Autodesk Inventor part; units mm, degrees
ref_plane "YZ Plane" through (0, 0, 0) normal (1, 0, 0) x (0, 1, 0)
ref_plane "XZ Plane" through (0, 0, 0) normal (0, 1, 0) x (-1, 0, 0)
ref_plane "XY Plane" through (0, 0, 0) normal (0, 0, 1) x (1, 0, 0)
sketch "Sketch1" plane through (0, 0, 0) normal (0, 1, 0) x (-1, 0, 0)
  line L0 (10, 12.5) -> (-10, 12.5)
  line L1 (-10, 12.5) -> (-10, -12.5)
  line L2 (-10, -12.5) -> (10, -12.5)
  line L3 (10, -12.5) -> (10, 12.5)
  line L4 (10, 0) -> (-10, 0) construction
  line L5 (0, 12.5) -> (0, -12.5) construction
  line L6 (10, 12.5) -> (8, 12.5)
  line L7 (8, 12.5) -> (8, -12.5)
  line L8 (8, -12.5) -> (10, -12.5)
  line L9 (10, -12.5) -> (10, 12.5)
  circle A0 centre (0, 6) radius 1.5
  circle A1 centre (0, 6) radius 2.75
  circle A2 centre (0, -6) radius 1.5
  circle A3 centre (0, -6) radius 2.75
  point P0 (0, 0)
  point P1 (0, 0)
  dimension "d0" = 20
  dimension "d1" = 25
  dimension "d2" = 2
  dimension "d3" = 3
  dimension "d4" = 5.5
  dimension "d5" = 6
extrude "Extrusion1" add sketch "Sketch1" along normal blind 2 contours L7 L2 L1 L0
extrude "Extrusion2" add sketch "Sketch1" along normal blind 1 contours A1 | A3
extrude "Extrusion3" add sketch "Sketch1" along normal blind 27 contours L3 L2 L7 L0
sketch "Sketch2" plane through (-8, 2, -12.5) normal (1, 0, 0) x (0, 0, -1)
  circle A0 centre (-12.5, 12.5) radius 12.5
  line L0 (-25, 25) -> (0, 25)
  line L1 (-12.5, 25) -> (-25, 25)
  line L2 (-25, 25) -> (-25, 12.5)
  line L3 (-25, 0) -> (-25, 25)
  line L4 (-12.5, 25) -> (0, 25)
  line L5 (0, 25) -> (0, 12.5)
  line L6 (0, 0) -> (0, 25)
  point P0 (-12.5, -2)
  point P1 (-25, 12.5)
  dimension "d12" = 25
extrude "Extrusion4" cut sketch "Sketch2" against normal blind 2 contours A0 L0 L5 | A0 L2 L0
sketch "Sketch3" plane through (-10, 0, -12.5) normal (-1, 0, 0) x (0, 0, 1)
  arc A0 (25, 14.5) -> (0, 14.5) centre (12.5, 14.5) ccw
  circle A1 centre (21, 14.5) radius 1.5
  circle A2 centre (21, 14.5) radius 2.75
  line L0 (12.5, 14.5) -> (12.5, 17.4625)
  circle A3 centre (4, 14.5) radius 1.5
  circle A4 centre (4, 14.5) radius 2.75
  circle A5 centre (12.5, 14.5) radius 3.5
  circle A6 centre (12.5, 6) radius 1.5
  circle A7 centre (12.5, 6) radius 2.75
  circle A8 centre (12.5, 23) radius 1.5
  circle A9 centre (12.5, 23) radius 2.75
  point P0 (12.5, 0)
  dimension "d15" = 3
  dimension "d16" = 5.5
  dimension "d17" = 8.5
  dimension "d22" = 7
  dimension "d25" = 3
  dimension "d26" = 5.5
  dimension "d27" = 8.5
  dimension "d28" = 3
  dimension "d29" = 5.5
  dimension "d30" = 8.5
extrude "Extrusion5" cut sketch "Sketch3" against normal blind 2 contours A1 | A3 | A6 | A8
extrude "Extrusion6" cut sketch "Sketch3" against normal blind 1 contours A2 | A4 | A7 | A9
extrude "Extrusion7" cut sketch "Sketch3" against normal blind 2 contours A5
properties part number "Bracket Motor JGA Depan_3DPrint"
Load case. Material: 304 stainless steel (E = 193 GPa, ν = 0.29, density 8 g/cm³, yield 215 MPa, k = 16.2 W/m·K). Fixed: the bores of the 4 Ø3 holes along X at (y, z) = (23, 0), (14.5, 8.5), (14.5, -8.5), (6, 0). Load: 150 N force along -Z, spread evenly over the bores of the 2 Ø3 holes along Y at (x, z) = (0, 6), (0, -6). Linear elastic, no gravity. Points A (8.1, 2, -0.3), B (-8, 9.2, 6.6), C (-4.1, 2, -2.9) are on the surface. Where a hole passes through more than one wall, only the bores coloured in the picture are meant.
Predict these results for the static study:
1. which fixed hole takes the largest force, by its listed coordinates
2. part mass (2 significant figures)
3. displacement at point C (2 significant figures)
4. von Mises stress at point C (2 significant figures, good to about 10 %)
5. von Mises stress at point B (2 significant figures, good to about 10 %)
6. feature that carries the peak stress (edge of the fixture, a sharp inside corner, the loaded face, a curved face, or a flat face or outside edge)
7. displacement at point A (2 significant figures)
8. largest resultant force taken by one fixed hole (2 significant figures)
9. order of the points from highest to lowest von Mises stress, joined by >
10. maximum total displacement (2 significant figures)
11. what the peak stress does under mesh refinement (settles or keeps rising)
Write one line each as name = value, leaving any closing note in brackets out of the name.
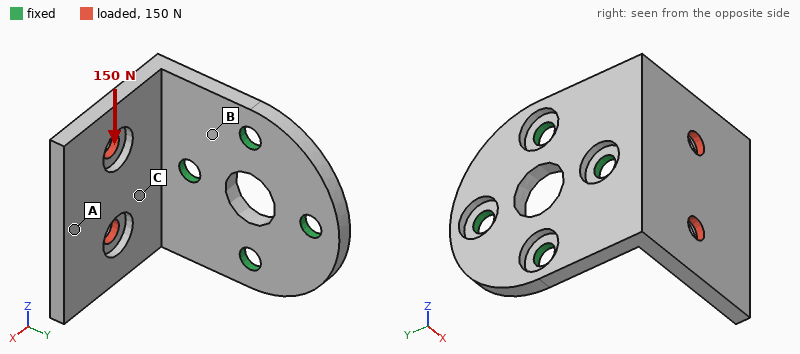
which fixed hole takes the largest force, by its listed coordinates = (6, 0)
part mass = 15 g
displacement at point C = 9.3 µm
von Mises stress at point C = 24 MPa
von Mises stress at point B = 38 MPa
feature that carries the peak stress = edge of the fixture
displacement at point A = 28 µm
largest resultant force taken by one fixed hole = 210 N
order of the points from highest to lowest von Mises stress, joined by > = B > C > A
maximum total displacement = 37 µm
what the peak stress does under mesh refinement = keeps rising
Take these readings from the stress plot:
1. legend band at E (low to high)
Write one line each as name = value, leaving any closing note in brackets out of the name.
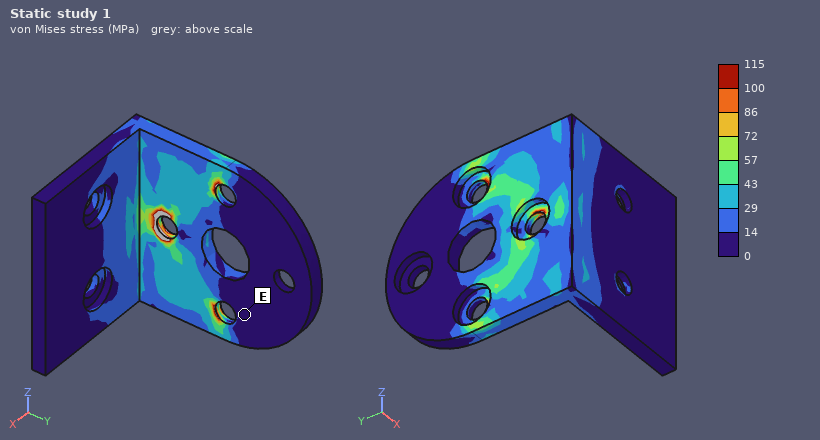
legend band at E = 0 to 14 MPa
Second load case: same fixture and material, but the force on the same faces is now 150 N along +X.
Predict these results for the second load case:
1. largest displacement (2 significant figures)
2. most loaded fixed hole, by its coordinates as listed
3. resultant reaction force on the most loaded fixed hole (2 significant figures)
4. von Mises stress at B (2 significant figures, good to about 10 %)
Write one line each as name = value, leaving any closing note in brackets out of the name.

largest displacement = 29 µm
most loaded fixed hole, by its coordinates as listed = (6, 0)
resultant reaction force on the most loaded fixed hole = 210 N
von Mises stress at B = 15 MPa
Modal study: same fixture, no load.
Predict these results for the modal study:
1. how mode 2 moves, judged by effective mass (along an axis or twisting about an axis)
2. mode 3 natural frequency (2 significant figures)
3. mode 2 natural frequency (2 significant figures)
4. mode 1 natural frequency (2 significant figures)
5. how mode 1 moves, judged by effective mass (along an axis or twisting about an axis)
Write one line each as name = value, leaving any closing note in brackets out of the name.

how mode 2 moves, judged by effective mass = along Z
mode 3 natural frequency = 7700 Hz
mode 2 natural frequency = 3900 Hz
mode 1 natural frequency = 2800 Hz
how mode 1 moves, judged by effective mass = along Y
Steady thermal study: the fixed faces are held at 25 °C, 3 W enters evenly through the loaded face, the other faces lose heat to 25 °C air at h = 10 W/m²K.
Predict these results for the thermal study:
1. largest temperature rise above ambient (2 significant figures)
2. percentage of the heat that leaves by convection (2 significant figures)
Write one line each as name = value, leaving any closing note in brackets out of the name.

largest temperature rise above ambient = 68 K
percentage of the heat that leaves by convection = 20 %
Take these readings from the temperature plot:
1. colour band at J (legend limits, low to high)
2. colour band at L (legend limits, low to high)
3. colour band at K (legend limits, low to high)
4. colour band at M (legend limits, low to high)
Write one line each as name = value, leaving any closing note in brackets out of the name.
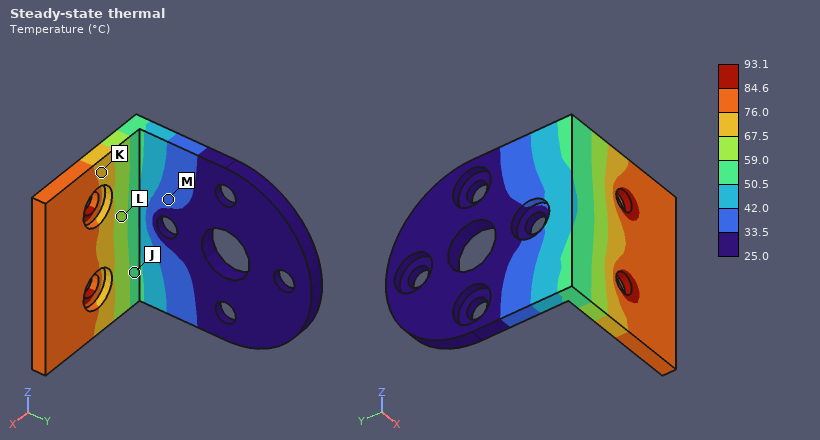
colour band at J = 50.5 to 59.0 °C
colour band at L = 59.0 to 67.5 °C
colour band at K = 67.5 to 76.0 °C
colour band at M = 33.5 to 42.0 °C
